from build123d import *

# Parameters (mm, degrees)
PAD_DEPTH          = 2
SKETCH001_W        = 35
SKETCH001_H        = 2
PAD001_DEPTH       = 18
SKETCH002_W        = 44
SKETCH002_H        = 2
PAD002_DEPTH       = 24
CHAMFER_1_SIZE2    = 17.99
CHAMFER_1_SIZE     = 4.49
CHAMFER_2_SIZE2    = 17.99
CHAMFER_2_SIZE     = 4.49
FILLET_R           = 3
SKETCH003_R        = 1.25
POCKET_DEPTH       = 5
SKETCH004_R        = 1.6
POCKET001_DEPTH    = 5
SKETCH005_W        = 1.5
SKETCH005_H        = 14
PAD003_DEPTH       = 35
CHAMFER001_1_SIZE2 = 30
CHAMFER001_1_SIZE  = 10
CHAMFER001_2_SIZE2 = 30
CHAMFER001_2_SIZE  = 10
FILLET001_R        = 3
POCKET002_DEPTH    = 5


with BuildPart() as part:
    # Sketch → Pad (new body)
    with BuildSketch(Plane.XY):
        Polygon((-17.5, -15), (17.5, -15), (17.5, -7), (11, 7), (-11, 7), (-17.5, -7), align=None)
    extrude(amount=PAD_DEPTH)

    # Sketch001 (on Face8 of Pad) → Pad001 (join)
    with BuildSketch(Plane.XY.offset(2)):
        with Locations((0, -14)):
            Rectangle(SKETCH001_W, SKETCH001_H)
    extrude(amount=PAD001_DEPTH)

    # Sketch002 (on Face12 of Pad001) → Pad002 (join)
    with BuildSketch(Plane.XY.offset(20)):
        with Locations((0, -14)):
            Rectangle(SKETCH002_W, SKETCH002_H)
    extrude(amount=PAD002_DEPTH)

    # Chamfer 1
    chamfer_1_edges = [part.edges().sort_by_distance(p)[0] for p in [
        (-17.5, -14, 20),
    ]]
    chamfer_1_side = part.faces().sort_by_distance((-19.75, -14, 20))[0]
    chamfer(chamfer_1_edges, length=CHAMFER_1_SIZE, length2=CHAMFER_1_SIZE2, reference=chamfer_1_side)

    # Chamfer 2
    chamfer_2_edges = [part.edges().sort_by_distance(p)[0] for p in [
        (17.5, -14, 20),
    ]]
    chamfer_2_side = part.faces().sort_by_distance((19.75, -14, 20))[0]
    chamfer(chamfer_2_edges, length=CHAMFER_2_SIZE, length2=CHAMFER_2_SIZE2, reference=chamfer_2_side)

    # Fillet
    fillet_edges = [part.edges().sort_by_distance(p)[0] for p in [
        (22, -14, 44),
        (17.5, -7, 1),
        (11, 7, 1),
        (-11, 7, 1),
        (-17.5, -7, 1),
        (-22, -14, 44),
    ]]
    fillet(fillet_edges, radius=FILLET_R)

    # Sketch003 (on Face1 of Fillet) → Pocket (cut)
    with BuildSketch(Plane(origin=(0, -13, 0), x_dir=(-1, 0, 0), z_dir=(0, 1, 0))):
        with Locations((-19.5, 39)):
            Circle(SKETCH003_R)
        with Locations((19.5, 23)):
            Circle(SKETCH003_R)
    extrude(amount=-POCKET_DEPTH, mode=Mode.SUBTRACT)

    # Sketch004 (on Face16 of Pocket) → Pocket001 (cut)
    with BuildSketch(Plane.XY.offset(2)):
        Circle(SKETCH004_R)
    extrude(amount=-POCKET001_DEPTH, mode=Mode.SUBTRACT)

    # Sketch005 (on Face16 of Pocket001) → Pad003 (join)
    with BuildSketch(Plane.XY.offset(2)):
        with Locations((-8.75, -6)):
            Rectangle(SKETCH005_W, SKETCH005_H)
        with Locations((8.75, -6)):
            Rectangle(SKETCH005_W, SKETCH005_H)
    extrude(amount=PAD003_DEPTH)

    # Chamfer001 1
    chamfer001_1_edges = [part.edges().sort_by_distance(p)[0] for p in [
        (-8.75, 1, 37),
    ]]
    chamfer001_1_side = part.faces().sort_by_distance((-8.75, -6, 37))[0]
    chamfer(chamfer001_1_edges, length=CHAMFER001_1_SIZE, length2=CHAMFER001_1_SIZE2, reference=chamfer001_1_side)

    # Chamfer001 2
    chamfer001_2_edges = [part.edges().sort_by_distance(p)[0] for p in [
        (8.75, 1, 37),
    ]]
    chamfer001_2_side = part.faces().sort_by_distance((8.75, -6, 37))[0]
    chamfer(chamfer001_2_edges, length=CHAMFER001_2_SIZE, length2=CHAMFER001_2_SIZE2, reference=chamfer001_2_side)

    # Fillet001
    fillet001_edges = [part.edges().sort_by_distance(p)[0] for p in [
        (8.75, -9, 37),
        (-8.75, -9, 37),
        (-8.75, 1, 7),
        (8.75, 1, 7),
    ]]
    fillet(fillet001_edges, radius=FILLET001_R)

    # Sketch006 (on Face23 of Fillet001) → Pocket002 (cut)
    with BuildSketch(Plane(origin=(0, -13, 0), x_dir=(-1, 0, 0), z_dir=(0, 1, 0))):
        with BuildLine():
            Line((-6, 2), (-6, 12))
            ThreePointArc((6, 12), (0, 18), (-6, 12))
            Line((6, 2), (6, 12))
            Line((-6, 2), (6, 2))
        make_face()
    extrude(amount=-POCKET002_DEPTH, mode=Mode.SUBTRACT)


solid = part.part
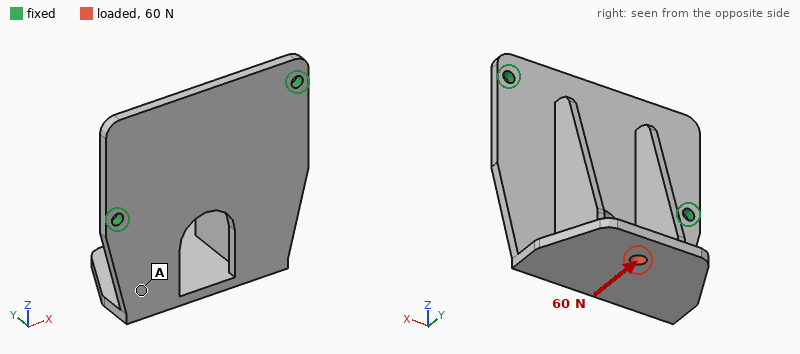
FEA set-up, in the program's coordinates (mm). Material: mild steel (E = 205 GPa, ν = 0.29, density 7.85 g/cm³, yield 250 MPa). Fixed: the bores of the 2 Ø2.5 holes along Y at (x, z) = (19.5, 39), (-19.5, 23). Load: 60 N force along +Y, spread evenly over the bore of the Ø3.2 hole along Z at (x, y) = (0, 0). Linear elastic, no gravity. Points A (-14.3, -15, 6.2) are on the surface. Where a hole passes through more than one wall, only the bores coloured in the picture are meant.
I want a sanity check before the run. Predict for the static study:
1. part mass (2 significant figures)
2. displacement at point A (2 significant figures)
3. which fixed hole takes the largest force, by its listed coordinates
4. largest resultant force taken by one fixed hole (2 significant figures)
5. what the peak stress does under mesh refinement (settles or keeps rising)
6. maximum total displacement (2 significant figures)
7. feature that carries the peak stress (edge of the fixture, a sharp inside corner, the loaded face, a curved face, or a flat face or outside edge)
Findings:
43 g
34 µm
(-19.5, 23)
49 N
keeps rising
100 µm
edge of the fixture
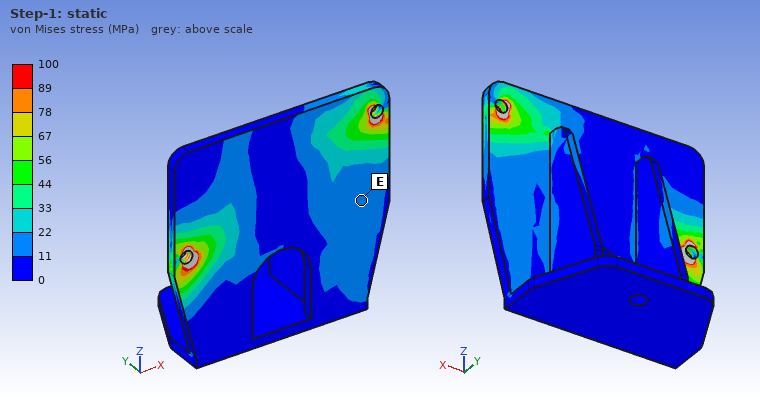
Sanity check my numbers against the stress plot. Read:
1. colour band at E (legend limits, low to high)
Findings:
11 to 22 MPa
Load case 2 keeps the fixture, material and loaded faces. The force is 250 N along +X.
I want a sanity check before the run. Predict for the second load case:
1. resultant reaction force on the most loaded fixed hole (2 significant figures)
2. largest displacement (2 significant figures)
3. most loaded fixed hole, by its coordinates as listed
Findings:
260 N
0.20 mm
(-19.5, 23)
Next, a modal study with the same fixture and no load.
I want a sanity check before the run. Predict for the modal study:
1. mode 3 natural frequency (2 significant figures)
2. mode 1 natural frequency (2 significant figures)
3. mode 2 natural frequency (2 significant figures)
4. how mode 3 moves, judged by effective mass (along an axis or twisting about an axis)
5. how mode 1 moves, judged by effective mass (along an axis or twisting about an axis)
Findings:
4600 Hz
1000 Hz
2700 Hz
along Y
along Y
